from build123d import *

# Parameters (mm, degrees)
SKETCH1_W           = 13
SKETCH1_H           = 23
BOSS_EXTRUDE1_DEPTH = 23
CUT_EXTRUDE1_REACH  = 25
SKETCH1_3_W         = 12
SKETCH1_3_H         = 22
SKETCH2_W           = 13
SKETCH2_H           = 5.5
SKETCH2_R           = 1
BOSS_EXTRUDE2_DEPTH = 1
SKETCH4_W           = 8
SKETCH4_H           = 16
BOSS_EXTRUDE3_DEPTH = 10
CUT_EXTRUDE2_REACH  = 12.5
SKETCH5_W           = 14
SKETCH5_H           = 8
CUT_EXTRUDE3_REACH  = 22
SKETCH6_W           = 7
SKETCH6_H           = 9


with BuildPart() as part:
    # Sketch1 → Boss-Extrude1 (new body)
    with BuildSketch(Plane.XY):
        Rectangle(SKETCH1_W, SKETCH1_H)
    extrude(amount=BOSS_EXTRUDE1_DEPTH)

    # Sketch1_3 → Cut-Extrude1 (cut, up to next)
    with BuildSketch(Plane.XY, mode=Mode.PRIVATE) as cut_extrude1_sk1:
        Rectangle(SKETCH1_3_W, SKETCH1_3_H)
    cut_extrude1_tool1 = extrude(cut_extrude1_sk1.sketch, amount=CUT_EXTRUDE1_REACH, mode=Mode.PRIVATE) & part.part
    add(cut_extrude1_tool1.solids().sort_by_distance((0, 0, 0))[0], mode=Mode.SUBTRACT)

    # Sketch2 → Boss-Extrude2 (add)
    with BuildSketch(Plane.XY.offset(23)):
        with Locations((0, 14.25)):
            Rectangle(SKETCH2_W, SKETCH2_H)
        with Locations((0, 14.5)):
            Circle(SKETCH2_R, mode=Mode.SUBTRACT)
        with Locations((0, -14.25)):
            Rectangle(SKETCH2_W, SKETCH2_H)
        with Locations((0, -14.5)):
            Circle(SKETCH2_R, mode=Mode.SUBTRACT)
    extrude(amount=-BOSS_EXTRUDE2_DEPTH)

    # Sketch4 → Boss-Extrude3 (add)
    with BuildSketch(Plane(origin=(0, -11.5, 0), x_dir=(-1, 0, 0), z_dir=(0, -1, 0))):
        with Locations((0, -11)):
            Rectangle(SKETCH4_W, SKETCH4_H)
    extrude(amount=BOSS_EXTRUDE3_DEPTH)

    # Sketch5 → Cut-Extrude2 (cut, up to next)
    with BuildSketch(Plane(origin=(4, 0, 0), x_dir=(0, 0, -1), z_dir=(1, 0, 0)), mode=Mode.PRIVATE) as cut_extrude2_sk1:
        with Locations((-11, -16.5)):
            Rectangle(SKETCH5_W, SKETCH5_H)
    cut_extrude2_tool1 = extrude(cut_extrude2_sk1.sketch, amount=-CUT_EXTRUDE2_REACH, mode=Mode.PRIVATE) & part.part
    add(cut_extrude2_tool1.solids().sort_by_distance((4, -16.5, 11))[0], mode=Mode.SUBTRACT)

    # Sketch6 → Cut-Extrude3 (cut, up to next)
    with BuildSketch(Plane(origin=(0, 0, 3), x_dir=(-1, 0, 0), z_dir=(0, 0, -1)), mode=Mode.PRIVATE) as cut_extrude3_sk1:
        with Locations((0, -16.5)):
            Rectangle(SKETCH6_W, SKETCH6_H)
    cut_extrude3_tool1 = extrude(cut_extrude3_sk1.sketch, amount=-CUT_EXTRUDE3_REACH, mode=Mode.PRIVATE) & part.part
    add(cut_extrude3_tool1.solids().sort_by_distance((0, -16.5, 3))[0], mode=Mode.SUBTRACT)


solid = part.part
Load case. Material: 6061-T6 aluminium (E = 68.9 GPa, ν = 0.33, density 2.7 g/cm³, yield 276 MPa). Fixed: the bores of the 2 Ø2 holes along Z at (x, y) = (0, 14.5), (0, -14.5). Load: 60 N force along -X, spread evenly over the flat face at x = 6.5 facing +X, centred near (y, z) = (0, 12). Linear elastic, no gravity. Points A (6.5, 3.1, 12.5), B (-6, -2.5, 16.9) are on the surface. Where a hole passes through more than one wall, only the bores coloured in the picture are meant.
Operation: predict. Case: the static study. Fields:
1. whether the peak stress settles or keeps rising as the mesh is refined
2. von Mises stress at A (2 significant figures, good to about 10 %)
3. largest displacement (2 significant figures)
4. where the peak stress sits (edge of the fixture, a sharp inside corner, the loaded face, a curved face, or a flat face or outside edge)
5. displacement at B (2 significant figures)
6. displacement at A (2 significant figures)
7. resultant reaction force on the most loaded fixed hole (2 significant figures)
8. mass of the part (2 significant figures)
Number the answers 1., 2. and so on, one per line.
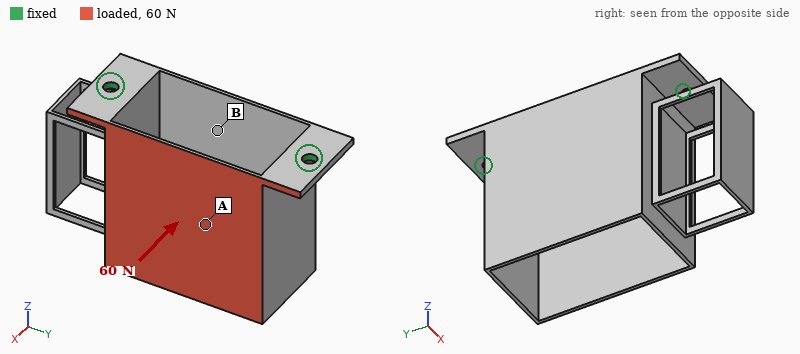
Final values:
1. keeps rising
2. 53 MPa
3. 0.38 mm
4. edge of the fixture
5. 0.066 mm
6. 0.22 mm
7. 31 N
8. 3.0 g
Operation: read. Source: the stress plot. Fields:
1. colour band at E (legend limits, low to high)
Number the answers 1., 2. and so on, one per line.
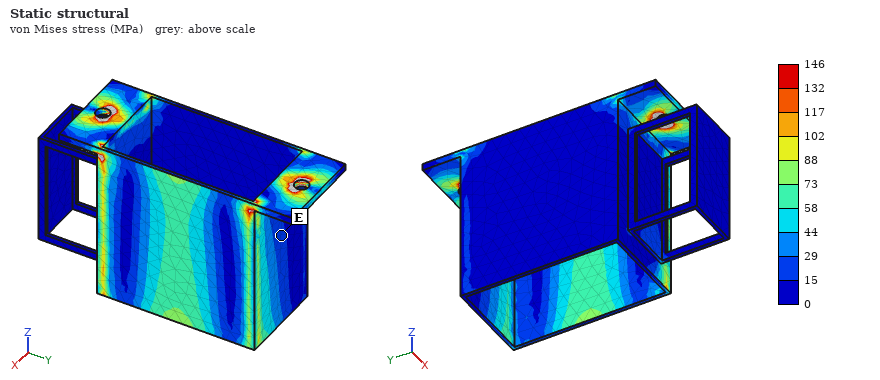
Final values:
1. 15 to 29 MPa
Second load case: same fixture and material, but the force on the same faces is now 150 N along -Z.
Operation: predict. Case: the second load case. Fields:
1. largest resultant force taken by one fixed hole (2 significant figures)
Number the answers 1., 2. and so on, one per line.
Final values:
1. 77 N
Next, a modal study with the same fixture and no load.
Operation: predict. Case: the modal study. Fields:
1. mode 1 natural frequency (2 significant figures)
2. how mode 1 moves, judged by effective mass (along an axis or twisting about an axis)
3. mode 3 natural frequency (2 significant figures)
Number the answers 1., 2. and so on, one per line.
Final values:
1. 1800 Hz
2. along X
3. 3400 Hz
